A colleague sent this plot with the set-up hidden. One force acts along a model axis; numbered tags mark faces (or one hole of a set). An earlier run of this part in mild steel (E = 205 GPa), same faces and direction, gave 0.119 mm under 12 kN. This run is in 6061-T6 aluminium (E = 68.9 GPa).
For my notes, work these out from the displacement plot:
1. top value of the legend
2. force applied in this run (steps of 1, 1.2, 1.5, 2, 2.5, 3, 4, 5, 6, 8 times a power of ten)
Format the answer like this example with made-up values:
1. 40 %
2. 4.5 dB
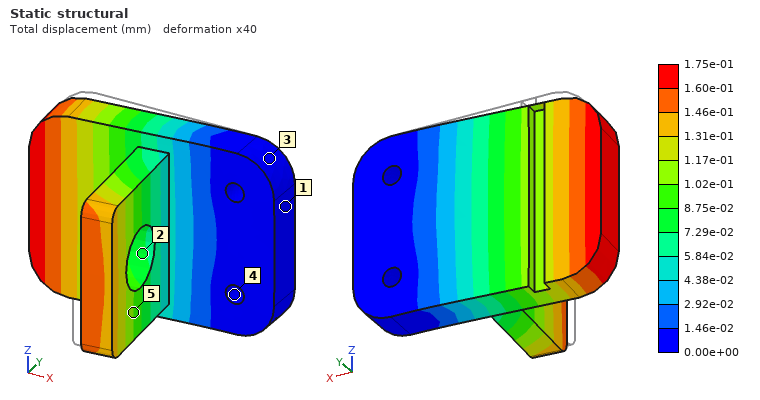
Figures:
1. 1.75e-01 mm
2. 6 kN
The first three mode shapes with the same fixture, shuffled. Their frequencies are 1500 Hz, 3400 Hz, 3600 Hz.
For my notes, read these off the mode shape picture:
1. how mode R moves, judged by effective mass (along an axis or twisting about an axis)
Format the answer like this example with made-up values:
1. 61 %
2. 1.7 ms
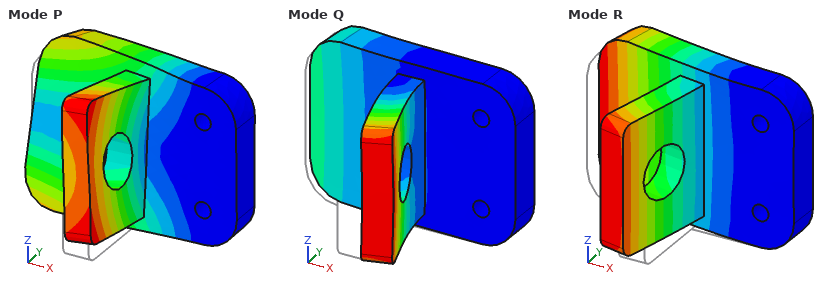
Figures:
1. along Y
